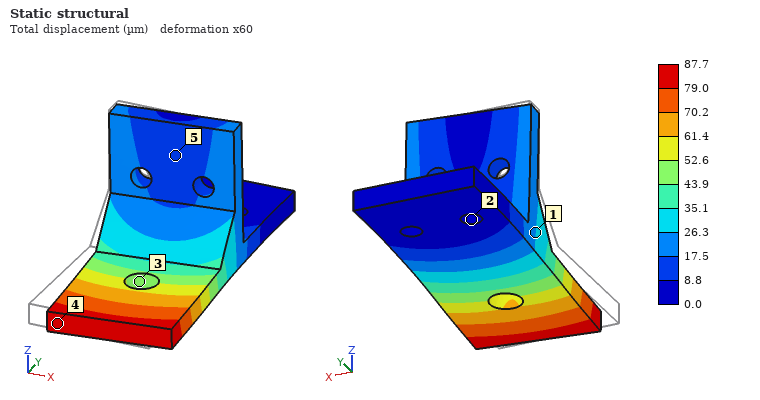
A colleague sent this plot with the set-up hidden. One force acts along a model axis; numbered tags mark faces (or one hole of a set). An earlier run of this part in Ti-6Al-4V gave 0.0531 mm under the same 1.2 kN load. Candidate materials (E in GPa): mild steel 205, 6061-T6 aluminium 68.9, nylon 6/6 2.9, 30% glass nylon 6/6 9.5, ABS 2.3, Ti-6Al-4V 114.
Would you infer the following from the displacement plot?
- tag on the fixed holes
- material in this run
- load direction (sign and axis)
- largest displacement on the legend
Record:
2
6061-T6 aluminium
+X
87.7 µm
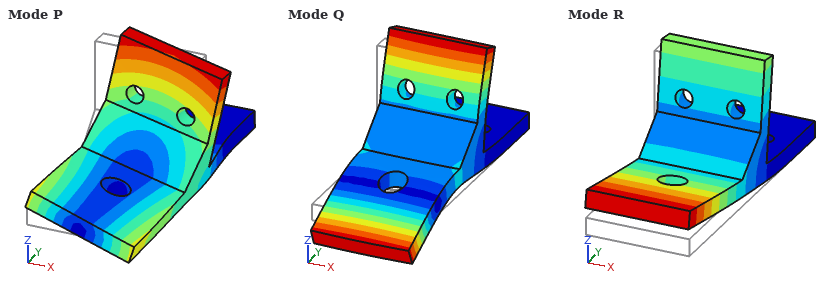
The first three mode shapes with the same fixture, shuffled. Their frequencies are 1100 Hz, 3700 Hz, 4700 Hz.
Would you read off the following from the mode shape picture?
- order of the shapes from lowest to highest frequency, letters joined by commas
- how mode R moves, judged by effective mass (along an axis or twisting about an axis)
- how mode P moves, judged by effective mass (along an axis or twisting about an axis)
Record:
R, P, Q
along Z
along X
